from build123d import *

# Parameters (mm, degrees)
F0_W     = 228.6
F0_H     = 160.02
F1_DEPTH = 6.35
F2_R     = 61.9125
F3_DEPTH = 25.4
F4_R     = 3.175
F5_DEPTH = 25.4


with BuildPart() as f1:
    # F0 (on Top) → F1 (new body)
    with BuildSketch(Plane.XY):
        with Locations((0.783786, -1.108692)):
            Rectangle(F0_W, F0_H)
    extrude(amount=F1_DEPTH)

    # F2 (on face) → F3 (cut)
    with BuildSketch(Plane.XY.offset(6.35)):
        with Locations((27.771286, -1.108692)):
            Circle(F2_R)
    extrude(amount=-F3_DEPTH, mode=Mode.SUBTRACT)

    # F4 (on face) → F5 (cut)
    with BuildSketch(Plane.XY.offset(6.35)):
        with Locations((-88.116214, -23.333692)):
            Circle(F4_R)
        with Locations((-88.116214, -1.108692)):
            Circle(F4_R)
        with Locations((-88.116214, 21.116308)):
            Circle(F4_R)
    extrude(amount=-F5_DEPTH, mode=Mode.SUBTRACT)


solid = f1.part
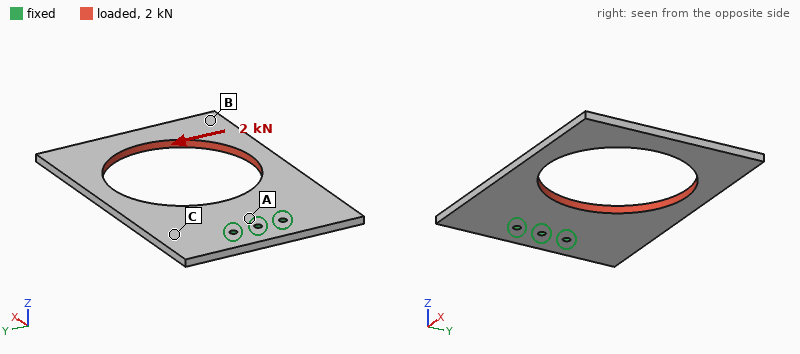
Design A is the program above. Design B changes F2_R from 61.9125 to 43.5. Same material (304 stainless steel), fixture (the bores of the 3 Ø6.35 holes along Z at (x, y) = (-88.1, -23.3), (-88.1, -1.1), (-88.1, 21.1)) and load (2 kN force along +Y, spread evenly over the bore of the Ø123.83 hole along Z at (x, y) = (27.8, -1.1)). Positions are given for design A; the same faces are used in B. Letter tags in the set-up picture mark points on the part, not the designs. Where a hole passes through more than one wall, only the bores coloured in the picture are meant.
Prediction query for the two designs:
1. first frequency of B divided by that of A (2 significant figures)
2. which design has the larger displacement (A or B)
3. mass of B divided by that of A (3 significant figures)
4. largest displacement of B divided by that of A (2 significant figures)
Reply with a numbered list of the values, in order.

1. 1.1
2. A
3. 1.25
4. 0.58
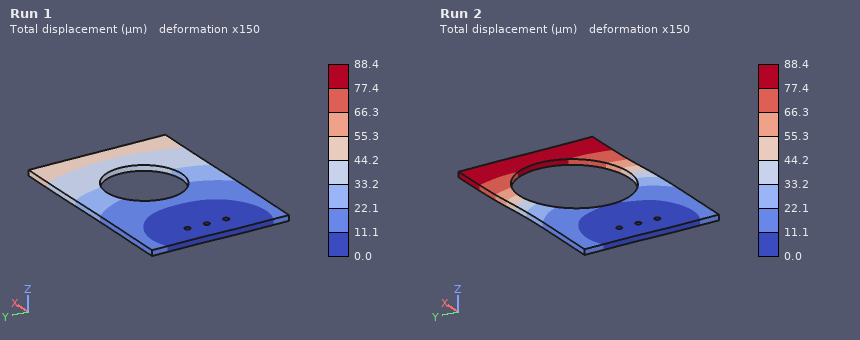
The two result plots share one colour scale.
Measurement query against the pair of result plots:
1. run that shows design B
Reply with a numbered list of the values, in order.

1. Run 1
